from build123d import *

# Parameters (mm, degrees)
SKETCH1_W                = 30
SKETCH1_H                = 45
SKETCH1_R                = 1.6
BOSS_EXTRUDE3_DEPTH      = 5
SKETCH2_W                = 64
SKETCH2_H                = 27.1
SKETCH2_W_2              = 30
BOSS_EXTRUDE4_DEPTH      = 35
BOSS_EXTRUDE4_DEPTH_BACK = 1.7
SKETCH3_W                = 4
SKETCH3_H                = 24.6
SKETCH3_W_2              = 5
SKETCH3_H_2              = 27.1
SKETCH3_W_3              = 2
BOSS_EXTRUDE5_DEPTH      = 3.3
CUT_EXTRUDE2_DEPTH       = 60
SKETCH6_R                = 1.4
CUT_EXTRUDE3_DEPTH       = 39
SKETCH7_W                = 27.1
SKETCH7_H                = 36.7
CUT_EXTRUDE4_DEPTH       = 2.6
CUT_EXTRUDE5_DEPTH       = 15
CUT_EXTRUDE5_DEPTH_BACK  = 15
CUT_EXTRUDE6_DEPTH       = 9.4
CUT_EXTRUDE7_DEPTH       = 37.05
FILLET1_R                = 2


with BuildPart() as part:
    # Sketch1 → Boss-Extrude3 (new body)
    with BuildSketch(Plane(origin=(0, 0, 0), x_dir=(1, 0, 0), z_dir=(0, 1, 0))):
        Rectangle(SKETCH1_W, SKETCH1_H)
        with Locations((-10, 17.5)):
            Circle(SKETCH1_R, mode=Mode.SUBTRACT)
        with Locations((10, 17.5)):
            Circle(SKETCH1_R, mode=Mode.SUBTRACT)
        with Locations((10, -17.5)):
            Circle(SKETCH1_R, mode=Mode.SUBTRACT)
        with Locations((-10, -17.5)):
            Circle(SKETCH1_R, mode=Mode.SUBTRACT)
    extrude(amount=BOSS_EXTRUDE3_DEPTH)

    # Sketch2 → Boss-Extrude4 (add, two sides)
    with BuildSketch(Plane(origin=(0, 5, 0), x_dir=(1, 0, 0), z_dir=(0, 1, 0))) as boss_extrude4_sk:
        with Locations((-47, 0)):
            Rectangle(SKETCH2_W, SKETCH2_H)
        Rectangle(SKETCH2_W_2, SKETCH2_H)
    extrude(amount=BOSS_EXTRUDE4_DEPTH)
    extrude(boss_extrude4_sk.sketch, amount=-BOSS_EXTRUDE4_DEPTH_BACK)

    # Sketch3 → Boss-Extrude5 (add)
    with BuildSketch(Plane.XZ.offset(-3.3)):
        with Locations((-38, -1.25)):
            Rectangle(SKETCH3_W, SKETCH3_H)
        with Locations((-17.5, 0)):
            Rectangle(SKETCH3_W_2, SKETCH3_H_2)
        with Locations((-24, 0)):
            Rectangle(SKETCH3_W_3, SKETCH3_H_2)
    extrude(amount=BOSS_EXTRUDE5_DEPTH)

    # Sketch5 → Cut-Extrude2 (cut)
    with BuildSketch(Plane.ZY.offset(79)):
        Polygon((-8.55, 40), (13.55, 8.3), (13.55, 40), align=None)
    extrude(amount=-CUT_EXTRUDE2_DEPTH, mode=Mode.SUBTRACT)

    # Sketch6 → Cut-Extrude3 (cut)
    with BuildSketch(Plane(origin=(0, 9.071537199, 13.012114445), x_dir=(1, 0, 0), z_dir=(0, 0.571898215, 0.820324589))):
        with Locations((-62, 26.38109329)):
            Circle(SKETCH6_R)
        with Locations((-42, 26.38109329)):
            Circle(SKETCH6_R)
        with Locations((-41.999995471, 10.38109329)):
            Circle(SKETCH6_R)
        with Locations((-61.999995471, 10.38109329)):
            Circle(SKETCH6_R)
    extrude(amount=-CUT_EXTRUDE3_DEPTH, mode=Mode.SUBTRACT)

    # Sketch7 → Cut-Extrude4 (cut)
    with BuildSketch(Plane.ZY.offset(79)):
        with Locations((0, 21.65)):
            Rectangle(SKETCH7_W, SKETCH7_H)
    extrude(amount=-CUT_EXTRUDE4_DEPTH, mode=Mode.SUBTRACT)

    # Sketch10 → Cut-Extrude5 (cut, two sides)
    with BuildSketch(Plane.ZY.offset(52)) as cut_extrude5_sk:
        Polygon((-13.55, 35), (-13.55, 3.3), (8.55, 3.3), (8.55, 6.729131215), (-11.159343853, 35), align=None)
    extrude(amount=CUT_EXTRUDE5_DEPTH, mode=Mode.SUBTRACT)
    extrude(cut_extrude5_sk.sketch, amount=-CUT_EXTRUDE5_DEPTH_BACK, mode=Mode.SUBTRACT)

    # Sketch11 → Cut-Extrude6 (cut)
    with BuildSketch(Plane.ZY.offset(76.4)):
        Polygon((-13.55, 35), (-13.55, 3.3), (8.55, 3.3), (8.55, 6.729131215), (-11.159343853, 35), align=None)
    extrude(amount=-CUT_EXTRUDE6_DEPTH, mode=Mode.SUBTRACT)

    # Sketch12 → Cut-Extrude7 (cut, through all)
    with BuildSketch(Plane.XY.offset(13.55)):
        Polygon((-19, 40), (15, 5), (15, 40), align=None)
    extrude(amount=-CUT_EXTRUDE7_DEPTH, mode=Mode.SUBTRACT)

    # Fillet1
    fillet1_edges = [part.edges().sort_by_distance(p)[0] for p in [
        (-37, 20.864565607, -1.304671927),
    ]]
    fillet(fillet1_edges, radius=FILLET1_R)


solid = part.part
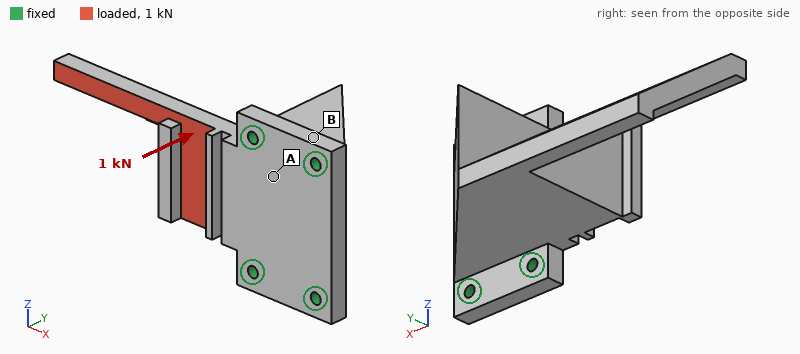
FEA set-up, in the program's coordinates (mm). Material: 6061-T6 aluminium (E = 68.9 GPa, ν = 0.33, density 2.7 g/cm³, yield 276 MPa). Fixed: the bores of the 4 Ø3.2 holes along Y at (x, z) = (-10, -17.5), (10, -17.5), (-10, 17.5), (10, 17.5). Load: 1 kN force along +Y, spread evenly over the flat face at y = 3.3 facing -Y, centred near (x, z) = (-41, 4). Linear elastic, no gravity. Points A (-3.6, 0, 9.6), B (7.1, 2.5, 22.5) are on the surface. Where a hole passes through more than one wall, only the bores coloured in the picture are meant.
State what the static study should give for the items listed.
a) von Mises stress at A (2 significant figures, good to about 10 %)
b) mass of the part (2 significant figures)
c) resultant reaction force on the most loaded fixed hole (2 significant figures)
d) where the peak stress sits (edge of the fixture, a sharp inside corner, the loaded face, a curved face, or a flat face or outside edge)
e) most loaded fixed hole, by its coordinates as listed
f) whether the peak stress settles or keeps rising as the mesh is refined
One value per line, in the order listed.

16 MPa
120 g
1.4 kN
edge of the fixture
(-10, 17.5)
keeps rising
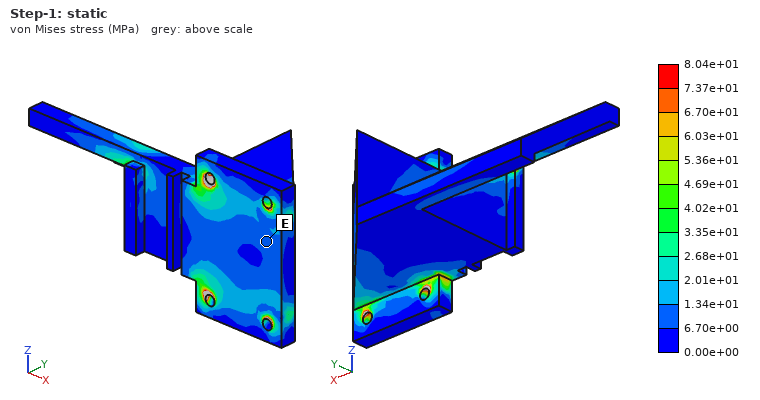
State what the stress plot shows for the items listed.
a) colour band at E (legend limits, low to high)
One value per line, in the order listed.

6.70e+00 to 1.34e+01 MPa
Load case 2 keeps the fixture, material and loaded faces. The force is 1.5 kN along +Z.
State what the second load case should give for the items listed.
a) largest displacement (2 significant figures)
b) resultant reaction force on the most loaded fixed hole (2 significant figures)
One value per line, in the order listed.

0.26 mm
1.2 kN
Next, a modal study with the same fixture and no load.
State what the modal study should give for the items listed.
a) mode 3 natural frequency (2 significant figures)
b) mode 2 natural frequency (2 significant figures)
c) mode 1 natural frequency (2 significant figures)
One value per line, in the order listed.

4900 Hz
3000 Hz
2100 Hz
